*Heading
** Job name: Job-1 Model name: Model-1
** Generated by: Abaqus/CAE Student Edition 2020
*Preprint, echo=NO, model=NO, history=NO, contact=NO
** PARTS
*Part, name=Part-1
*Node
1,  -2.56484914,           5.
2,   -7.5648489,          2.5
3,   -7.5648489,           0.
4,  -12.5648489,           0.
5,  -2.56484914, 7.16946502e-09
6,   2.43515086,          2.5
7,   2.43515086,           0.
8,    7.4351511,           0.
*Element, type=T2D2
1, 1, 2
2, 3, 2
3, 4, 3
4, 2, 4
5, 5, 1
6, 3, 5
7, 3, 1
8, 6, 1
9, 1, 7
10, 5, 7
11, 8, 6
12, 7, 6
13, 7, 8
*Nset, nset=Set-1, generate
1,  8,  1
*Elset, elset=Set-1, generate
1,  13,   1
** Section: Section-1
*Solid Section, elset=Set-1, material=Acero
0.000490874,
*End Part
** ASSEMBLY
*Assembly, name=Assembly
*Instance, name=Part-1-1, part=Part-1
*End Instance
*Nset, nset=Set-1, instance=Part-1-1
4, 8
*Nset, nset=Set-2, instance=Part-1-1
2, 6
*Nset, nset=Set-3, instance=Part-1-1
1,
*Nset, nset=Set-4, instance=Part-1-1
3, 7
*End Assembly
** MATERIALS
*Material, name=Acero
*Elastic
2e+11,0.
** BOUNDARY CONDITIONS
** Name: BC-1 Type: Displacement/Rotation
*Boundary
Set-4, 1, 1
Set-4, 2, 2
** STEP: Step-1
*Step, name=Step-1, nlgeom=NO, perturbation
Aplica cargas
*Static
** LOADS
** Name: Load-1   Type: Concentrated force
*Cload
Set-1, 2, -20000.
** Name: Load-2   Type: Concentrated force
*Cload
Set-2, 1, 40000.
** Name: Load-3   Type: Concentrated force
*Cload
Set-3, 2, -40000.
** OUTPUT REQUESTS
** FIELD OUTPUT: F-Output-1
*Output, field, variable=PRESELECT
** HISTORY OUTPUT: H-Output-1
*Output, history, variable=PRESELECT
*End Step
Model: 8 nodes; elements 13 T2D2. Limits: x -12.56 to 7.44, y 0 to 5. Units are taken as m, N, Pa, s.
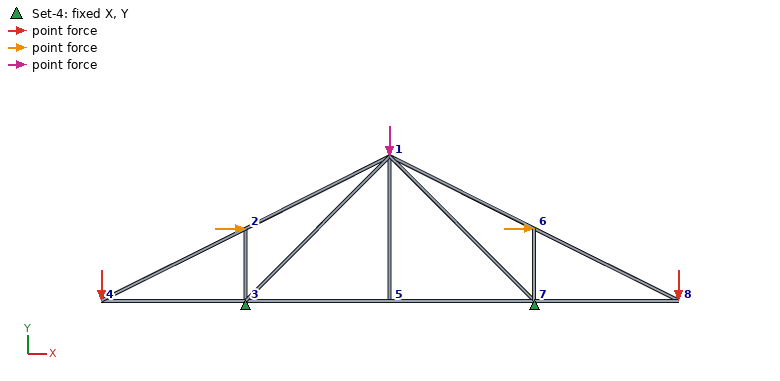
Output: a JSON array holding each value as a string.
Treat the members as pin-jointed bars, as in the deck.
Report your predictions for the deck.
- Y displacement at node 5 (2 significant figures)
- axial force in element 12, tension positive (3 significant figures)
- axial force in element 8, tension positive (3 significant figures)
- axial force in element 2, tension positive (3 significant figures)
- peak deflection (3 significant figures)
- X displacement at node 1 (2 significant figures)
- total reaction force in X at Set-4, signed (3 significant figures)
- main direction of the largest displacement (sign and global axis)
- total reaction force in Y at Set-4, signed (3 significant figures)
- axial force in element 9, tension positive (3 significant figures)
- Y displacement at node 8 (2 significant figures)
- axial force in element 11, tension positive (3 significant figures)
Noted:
["-0.0058 m", "20000 N", "89400 N", "-20000 N", "0.0385 m", "0.0058 m", "-80000 N", "-Y", "80000 N", "-1.13e+05 N", "-0.038 m", "44700 N"]
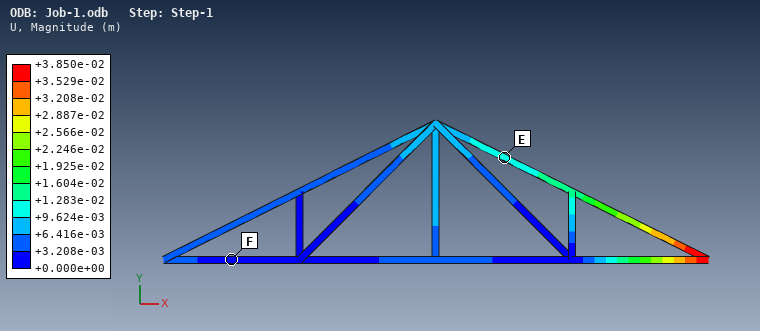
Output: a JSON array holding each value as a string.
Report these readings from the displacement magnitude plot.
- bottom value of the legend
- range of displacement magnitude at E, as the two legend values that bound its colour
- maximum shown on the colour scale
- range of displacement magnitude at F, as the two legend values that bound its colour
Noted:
["+0.000e+00 m", "+9.624e-03 to +1.283e-02 m", "+3.850e-02 m", "+0.000e+00 to +3.208e-03 m"]
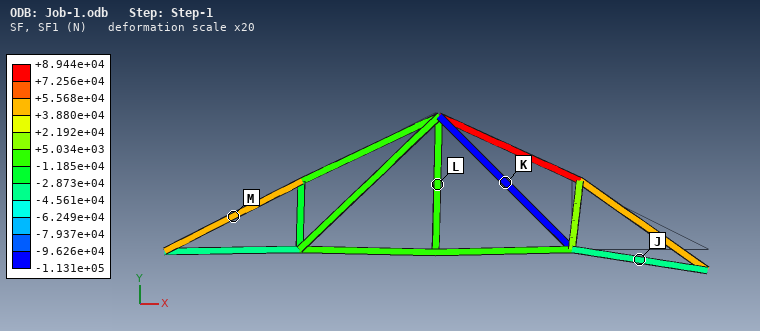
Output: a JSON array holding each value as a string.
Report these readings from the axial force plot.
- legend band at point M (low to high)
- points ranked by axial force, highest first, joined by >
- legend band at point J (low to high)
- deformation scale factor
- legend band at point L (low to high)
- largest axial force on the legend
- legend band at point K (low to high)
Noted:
["+3.880e+04 to +5.568e+04 N", "M > L > J > K", "-4.561e+04 to -2.873e+04 N", "20", "-1.185e+04 to +5.034e+03 N", "+8.944e+04 N", "-1.131e+05 to -9.626e+04 N"]
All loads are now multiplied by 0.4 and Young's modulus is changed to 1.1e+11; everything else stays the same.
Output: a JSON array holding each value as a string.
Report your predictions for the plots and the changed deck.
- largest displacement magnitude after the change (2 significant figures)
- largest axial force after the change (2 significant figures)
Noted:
["0.028 m", "36000 N"]
